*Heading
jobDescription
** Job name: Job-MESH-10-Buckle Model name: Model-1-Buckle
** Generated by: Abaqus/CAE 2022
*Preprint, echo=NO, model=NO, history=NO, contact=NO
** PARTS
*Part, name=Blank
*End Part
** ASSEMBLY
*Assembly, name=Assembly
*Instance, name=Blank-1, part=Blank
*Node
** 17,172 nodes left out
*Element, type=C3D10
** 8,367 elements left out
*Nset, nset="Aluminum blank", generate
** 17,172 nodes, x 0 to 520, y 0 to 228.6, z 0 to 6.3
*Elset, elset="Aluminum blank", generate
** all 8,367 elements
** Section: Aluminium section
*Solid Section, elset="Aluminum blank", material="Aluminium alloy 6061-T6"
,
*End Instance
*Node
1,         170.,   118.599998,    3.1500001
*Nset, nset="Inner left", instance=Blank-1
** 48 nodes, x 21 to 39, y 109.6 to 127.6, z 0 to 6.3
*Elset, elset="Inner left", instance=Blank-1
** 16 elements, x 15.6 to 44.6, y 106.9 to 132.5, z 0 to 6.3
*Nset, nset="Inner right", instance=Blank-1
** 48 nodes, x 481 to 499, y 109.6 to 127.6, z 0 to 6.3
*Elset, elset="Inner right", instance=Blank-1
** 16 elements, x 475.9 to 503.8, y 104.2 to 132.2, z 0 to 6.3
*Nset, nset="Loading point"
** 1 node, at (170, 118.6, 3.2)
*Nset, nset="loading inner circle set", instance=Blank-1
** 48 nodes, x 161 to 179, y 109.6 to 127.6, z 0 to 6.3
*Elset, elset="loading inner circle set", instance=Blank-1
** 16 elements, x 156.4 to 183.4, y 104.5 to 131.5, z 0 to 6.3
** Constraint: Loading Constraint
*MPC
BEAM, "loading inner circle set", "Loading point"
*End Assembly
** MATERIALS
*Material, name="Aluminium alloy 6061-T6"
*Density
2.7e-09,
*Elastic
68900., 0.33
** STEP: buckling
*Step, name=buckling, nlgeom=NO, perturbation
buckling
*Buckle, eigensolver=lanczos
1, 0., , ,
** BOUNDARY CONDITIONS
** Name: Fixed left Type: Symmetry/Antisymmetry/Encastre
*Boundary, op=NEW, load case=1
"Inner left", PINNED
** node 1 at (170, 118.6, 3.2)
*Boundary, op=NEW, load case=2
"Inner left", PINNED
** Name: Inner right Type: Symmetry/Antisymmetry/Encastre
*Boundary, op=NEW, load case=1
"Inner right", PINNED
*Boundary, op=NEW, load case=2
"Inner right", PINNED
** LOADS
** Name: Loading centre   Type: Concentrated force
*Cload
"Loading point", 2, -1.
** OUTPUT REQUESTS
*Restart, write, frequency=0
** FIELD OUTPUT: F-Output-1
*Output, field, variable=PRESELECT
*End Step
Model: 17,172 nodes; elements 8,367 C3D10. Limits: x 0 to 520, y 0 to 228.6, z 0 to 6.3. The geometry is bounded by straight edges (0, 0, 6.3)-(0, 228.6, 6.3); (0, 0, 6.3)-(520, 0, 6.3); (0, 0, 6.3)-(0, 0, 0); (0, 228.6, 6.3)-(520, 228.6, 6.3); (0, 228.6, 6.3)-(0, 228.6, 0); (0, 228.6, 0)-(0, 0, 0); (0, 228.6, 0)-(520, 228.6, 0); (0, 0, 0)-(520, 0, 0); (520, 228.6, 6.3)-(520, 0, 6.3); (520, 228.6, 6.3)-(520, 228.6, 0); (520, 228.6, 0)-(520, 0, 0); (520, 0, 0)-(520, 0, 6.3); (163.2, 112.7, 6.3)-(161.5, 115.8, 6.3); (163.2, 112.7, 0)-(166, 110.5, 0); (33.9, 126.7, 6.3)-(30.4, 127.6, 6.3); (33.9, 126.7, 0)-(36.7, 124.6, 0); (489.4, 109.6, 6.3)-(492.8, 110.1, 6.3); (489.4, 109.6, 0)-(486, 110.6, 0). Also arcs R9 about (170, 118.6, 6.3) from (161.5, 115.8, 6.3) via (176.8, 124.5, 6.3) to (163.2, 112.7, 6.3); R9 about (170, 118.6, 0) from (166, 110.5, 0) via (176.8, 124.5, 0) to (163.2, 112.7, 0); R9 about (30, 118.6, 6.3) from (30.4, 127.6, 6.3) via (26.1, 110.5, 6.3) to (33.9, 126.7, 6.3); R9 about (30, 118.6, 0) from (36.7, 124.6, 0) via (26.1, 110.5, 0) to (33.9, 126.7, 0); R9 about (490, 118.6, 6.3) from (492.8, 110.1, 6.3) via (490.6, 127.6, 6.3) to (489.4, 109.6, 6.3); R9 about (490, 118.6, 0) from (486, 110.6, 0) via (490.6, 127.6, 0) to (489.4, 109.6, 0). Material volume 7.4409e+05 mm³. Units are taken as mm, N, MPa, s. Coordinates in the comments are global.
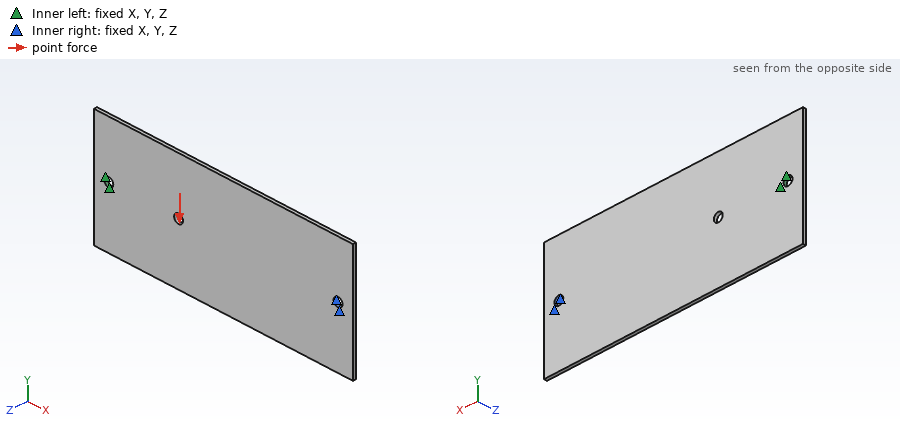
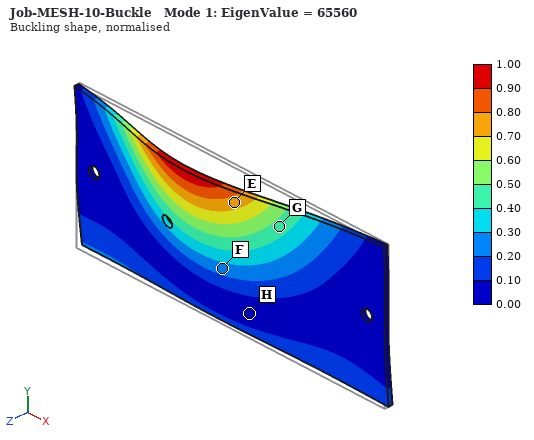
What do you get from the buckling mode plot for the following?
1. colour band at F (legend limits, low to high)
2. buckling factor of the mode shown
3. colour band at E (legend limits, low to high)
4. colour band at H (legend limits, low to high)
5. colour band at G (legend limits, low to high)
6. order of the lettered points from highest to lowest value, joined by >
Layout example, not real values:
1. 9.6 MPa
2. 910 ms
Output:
1. 0.20 to 0.30
2. 65560
3. 0.70 to 0.80
4. 0.00 to 0.10
5. 0.40 to 0.50
6. E > G > F > H
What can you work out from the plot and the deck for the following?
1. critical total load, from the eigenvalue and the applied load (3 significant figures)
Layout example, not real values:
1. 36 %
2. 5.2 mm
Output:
1. 65600 N
